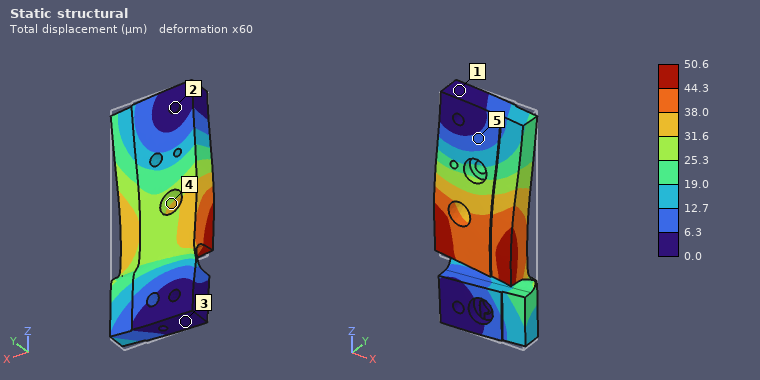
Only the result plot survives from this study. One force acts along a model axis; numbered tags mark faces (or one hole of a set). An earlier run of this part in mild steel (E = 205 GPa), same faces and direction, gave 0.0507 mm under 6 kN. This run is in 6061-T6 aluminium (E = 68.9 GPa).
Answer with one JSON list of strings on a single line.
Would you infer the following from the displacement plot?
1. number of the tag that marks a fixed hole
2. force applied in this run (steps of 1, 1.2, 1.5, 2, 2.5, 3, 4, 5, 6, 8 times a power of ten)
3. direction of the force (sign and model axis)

["2", "2 kN", "-X"]
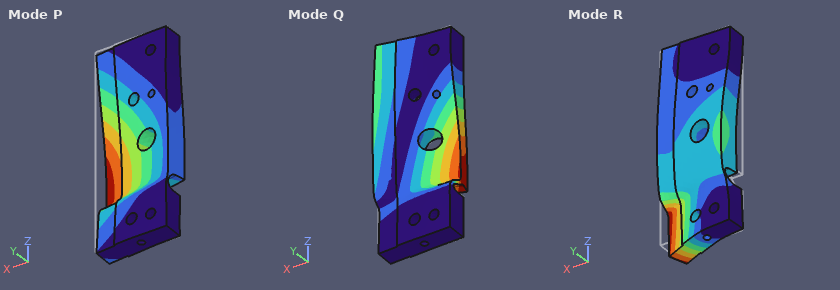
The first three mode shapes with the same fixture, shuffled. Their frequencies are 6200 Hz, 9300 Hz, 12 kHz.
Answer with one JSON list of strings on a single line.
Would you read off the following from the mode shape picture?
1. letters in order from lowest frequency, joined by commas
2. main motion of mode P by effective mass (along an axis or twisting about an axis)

["P, Q, R", "along Y"]
